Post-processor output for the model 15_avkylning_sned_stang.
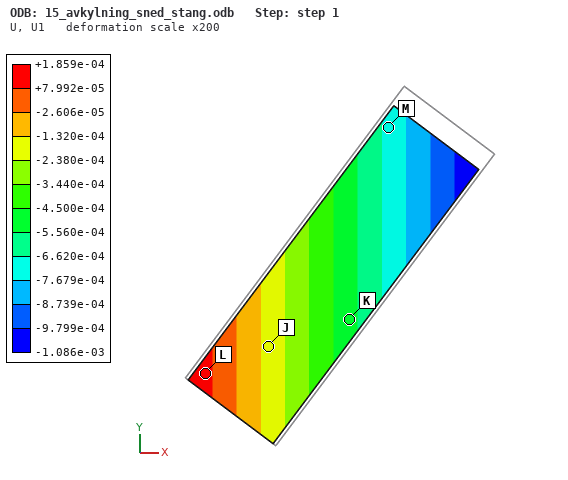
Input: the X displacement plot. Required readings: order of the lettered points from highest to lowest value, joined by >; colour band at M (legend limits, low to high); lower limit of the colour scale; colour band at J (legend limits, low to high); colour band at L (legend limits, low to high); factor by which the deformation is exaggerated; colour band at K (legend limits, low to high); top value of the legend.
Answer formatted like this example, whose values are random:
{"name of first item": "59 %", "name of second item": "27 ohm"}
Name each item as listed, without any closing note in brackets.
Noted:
{"order of the lettered points from highest to lowest value, joined by >": "L > J > K > M", "colour band at M": "-7.679e-04 to -6.620e-04", "lower limit of the colour scale": "-1.086e-03", "colour band at J": "-2.380e-04 to -1.320e-04", "colour band at L": "+7.992e-05 to +1.859e-04", "factor by which the deformation is exaggerated": "200", "colour band at K": "-5.560e-04 to -4.500e-04", "top value of the legend": "+1.859e-04"}
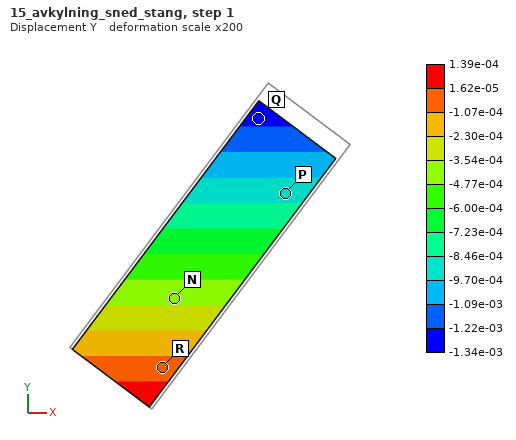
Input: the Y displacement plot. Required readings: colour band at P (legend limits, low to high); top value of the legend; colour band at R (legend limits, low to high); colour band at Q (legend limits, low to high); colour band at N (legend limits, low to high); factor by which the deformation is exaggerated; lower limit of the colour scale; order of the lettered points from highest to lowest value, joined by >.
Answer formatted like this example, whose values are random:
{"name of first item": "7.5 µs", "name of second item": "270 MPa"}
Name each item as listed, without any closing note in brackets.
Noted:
{"colour band at P": "-9.70e-04 to -8.46e-04", "top value of the legend": "1.39e-04", "colour band at R": "-1.07e-04 to 1.62e-05", "colour band at Q": "-1.34e-03 to -1.22e-03", "colour band at N": "-4.77e-04 to -3.54e-04", "factor by which the deformation is exaggerated": "200", "lower limit of the colour scale": "-1.34e-03", "order of the lettered points from highest to lowest value, joined by >": "R > N > P > Q"}
